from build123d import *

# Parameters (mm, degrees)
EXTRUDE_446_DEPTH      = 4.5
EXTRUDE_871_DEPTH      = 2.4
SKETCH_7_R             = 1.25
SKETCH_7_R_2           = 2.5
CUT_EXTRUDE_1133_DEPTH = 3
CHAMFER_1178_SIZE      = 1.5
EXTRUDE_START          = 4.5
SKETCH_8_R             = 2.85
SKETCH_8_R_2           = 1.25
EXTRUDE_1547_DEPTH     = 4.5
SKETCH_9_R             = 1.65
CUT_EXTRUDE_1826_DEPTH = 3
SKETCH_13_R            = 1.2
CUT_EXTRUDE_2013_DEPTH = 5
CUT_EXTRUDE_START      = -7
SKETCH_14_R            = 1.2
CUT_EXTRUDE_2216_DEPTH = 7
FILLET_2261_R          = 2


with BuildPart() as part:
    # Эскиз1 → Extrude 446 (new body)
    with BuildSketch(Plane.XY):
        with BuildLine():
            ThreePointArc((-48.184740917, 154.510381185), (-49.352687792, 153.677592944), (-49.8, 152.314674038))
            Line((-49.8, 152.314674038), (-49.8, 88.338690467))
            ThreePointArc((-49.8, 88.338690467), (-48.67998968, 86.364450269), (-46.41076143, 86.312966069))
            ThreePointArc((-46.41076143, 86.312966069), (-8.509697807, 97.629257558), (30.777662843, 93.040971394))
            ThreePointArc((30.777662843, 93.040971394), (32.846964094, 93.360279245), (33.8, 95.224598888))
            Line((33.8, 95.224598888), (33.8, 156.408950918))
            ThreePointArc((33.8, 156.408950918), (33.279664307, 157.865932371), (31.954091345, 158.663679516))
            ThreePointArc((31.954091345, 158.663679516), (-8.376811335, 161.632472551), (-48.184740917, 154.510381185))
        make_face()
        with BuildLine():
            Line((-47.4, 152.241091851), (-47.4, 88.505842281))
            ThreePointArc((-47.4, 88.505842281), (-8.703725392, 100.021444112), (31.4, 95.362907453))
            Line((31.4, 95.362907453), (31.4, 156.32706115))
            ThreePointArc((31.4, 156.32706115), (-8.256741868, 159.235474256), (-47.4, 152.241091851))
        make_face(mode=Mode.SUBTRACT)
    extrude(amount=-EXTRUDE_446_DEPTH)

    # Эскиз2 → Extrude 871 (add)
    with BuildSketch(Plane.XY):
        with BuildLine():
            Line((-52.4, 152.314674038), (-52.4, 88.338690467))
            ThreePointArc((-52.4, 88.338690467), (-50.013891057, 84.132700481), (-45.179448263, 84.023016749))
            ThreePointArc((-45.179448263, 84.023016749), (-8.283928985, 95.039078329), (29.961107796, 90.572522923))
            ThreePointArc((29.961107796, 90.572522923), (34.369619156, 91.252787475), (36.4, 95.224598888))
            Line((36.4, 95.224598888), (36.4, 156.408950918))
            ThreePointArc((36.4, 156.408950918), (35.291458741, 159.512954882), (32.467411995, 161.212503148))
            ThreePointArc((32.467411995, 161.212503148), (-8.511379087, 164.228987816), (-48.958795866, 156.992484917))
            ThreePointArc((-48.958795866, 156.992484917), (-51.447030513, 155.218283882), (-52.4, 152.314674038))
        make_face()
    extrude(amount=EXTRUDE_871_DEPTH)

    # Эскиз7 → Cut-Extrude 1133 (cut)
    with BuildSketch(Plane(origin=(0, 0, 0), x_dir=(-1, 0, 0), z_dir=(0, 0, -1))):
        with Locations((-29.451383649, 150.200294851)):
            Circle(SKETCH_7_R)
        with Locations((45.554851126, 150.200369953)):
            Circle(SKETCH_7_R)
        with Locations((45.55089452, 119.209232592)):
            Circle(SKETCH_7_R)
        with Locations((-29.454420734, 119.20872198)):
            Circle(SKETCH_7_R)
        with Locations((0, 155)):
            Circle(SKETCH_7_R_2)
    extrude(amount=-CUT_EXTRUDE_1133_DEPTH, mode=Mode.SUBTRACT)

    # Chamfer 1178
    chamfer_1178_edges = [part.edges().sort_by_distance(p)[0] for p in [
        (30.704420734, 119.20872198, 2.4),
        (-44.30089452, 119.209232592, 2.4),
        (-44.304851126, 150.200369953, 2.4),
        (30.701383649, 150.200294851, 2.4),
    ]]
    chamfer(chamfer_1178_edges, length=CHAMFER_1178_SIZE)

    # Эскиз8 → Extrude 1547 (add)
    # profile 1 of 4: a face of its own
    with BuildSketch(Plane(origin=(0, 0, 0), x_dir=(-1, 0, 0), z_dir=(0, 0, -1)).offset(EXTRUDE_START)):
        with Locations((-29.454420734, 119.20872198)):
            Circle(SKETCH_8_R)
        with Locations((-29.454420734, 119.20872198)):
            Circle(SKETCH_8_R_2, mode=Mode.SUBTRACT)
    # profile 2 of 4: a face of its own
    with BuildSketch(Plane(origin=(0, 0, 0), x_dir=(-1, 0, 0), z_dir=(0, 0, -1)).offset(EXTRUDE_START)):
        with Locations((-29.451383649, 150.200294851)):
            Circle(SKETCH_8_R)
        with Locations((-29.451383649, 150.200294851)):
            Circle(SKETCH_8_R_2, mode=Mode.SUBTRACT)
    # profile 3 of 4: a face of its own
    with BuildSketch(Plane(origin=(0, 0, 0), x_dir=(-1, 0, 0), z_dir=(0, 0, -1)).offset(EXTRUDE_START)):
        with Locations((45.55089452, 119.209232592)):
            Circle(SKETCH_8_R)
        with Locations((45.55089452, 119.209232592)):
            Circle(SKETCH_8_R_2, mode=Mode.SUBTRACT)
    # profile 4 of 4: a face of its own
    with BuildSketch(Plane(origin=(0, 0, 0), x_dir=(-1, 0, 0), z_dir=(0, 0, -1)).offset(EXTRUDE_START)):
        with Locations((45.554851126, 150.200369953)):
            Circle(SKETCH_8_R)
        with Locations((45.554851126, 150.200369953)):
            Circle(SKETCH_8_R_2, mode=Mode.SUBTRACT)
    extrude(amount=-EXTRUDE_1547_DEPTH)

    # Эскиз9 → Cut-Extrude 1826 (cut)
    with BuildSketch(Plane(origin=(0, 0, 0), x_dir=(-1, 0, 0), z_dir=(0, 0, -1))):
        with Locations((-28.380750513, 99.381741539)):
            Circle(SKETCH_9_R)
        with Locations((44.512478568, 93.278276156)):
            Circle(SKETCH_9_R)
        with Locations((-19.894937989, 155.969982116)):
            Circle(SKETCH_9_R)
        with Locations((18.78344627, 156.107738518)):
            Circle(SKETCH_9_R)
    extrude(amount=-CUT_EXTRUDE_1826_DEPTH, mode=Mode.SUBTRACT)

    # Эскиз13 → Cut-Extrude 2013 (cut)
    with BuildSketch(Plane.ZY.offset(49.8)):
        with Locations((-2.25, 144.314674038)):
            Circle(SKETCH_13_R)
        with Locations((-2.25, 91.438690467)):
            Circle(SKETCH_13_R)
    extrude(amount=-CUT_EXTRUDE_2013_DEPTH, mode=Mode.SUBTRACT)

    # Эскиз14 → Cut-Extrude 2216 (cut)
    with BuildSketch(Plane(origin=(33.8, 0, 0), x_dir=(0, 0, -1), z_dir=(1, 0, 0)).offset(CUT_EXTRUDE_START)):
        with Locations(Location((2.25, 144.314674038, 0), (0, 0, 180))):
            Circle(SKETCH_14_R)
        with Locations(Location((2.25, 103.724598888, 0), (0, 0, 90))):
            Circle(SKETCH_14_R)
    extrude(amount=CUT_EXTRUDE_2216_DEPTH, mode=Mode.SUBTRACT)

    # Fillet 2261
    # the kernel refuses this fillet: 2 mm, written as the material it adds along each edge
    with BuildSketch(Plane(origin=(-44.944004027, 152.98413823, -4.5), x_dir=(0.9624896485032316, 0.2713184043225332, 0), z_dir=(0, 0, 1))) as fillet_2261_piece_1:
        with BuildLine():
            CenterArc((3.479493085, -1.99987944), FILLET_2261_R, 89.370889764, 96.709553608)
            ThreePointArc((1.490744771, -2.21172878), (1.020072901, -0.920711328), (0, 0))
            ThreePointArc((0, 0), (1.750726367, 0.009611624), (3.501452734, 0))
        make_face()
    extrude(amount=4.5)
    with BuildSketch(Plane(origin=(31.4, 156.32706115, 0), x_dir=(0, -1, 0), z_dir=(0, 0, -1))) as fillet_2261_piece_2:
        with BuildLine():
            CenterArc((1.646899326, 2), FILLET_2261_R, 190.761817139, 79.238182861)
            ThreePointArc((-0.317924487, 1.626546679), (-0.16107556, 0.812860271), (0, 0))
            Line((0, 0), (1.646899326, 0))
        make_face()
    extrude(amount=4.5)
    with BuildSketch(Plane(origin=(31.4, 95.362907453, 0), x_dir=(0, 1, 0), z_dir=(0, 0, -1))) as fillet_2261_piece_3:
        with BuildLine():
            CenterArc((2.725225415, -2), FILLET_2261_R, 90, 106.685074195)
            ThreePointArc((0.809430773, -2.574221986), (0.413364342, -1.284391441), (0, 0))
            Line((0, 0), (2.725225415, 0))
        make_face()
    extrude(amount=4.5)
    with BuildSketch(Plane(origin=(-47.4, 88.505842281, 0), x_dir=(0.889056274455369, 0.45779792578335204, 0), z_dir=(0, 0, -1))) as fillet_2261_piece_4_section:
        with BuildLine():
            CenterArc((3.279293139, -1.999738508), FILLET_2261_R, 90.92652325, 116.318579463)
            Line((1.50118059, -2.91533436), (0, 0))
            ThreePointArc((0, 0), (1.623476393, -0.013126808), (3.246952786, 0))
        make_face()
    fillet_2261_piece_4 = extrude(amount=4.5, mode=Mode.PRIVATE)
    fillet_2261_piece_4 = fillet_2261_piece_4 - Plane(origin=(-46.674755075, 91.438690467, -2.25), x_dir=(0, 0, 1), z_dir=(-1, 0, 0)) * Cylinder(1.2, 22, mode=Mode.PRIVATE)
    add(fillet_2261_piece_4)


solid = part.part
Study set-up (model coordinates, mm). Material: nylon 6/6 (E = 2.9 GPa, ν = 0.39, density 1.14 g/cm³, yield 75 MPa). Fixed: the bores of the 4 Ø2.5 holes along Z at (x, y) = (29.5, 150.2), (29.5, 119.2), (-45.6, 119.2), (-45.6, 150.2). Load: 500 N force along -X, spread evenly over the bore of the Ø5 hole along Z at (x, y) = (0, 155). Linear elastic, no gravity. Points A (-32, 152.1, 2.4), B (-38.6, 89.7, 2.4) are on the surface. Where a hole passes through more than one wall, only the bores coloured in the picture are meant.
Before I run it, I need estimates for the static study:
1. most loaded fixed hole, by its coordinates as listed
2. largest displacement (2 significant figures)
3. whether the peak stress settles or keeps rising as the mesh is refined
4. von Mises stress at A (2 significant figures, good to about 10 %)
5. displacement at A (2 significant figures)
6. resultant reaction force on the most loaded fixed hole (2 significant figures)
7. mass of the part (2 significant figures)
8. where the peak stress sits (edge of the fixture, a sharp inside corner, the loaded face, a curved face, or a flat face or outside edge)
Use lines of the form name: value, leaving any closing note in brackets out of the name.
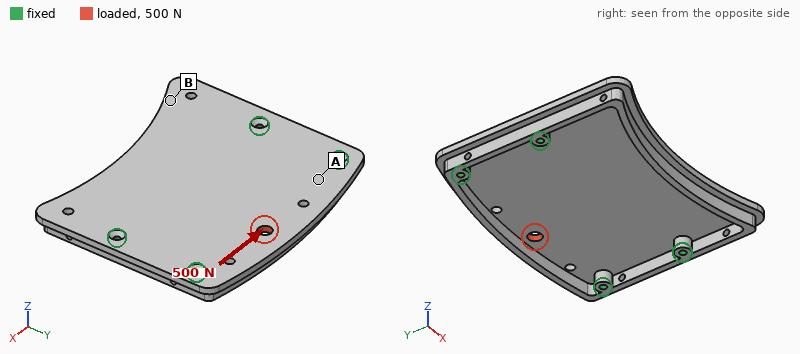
most loaded fixed hole, by its coordinates as listed: (29.5, 150.2)
largest displacement: 84 µm
whether the peak stress settles or keeps rising as the mesh is refined: keeps rising
von Mises stress at A: 2.8 MPa
displacement at A: 20 µm
resultant reaction force on the most loaded fixed hole: 220 N
mass of the part: 21 g
where the peak stress sits: edge of the fixture
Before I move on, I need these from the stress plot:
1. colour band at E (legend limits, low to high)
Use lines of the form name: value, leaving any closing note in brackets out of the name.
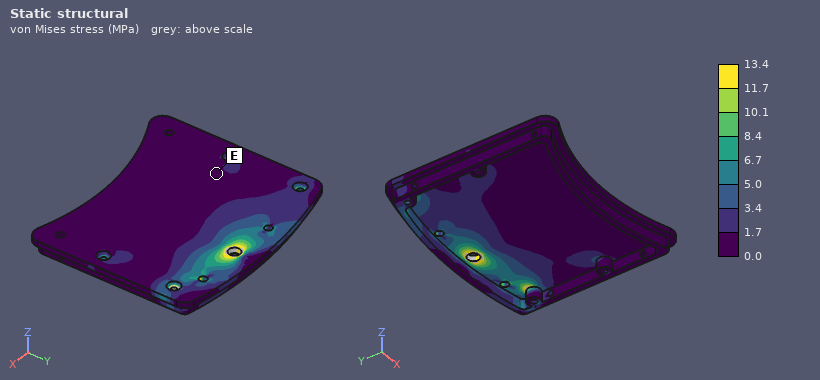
colour band at E: 0.0 to 1.7 MPa
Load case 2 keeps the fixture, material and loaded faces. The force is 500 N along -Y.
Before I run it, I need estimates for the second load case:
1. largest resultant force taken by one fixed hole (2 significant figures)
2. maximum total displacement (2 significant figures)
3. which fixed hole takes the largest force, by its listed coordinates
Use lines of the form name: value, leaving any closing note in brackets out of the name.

largest resultant force taken by one fixed hole: 170 N
maximum total displacement: 0.16 mm
which fixed hole takes the largest force, by its listed coordinates: (29.5, 119.2)
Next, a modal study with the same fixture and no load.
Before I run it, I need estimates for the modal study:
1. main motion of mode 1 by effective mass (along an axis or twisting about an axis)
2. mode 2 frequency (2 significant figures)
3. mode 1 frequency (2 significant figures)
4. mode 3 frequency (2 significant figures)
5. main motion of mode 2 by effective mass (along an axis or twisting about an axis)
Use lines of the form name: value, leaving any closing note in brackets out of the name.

main motion of mode 1 by effective mass: along Z
mode 2 frequency: 960 Hz
mode 1 frequency: 650 Hz
mode 3 frequency: 1200 Hz
main motion of mode 2 by effective mass: along Z
